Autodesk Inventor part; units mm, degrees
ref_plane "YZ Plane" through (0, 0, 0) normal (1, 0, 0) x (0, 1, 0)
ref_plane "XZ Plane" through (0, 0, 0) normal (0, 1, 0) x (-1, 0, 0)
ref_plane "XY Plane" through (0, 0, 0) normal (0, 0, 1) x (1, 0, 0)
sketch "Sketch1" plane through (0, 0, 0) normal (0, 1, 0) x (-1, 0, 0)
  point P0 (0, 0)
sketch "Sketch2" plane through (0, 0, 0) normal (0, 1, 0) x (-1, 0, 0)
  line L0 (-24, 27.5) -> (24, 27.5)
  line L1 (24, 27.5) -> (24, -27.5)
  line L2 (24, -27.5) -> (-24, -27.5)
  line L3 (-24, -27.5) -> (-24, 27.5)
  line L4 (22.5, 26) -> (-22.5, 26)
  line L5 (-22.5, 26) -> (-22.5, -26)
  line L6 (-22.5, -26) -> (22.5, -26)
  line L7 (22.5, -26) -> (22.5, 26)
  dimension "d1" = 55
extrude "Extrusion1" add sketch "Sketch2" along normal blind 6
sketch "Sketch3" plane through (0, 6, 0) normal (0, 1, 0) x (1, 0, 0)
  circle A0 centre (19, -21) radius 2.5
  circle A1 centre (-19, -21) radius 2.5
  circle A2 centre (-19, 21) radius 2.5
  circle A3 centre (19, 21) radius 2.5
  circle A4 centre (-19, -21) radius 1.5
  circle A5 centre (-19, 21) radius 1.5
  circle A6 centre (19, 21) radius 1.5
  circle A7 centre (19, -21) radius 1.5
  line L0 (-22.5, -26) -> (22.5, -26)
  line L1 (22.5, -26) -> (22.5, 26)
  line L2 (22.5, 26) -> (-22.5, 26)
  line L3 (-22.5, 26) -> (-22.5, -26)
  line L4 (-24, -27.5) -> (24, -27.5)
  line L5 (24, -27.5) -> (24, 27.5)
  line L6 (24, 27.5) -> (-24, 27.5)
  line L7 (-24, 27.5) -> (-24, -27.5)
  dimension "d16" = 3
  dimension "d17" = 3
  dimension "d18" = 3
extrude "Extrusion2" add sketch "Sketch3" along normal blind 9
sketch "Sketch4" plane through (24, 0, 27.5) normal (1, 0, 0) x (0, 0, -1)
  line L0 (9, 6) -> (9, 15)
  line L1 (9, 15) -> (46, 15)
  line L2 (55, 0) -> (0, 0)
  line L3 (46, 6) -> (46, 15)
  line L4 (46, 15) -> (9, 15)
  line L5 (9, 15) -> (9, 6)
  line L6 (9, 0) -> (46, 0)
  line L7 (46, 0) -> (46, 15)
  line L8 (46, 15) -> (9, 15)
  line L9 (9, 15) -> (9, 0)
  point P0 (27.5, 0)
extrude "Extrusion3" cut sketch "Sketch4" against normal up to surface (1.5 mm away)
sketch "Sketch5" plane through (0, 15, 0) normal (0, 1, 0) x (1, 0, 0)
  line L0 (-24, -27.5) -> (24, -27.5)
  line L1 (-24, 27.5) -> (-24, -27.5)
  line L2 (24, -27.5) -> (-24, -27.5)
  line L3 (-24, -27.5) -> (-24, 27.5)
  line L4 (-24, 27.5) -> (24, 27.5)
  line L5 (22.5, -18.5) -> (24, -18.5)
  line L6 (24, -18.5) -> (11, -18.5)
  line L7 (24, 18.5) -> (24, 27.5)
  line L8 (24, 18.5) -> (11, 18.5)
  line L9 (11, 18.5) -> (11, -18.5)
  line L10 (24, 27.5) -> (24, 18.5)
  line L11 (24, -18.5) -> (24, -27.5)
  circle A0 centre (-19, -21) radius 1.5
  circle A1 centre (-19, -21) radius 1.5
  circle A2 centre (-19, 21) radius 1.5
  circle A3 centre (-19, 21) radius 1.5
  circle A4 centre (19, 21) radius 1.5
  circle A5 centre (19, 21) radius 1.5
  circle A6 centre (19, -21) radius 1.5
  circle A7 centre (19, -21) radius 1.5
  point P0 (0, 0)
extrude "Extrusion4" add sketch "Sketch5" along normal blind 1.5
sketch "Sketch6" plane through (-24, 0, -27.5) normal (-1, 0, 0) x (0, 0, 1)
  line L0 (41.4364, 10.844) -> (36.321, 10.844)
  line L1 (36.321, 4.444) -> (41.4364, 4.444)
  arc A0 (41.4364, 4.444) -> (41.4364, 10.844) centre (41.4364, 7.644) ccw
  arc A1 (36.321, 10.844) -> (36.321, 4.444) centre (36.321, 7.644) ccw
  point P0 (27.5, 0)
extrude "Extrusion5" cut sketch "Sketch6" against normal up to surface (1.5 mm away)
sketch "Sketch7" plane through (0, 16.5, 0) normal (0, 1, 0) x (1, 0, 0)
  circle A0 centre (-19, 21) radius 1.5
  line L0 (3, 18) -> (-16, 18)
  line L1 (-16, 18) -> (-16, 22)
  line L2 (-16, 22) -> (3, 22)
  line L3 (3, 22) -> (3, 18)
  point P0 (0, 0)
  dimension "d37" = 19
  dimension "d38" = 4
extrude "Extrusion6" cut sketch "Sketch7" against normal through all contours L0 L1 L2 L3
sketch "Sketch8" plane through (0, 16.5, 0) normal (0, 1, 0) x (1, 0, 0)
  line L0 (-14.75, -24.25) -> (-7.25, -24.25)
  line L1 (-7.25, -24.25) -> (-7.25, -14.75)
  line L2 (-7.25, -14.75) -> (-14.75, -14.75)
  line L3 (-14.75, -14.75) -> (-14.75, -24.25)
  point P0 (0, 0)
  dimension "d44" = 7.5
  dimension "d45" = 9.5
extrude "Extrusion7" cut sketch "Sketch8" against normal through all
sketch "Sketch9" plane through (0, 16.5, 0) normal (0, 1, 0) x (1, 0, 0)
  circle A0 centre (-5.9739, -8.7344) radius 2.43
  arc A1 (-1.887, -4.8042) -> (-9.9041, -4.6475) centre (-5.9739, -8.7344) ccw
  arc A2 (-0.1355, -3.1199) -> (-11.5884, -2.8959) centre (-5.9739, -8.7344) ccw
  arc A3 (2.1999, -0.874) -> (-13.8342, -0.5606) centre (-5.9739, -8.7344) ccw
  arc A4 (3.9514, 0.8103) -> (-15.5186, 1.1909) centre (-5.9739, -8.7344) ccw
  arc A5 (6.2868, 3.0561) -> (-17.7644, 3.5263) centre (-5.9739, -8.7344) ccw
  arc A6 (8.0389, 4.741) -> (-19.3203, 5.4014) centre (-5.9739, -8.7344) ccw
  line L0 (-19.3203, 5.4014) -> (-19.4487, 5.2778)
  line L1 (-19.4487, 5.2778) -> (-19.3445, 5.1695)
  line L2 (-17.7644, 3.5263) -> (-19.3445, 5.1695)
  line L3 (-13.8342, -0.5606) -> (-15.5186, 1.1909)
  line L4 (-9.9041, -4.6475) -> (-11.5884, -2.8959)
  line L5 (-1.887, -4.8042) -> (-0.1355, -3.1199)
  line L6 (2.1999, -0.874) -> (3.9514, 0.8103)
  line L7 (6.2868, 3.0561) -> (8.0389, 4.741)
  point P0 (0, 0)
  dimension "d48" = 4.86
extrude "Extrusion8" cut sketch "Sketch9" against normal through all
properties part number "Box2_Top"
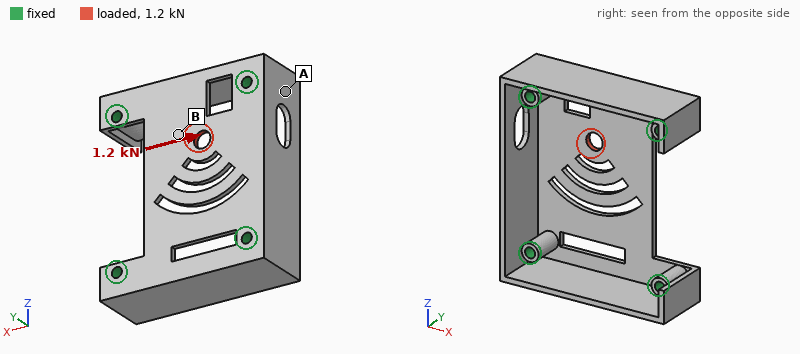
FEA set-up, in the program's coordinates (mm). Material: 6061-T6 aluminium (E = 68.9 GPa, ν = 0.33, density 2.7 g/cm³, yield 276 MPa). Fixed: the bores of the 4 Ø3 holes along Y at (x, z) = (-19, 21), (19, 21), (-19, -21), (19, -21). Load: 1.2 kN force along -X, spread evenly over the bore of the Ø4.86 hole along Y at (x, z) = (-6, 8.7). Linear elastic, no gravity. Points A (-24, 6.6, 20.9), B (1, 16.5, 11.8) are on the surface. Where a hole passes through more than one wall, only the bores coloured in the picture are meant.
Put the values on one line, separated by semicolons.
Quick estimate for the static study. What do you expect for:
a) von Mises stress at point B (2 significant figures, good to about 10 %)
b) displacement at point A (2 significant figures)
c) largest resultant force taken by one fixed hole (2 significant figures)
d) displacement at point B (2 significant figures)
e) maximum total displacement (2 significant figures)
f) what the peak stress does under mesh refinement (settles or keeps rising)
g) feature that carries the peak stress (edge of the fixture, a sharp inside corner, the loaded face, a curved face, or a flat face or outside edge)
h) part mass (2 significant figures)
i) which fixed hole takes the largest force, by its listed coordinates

35 MPa; 6.2 µm; 600 N; 19 µm; 27 µm; keeps rising; edge of the fixture; 18 g; (-19, 21)
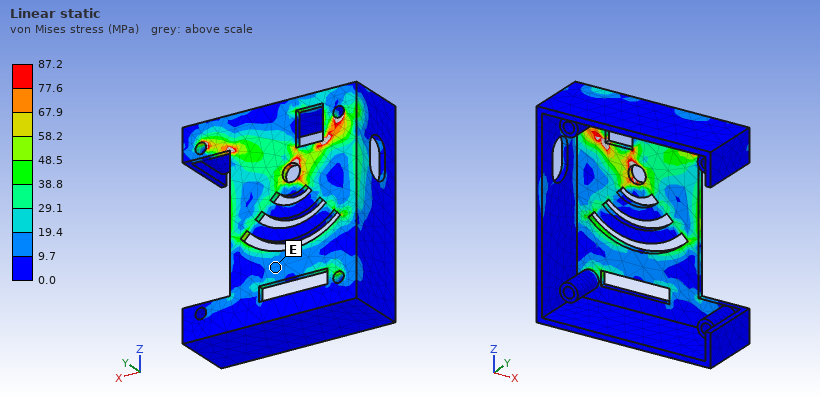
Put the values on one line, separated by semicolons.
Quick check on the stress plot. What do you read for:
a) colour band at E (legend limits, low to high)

9.7 to 19.4 MPa
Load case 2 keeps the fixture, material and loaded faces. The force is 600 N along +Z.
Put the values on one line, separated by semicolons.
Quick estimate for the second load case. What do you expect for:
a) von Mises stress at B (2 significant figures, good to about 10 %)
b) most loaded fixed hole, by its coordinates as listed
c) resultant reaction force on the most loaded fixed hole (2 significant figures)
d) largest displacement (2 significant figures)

18 MPa; (-19, 21); 320 N; 16 µm
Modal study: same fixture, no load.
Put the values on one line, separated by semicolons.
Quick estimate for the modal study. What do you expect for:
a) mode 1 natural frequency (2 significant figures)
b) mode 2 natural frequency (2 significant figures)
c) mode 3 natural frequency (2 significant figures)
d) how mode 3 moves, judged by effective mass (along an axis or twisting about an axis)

3000 Hz; 4300 Hz; 4500 Hz; along Z
